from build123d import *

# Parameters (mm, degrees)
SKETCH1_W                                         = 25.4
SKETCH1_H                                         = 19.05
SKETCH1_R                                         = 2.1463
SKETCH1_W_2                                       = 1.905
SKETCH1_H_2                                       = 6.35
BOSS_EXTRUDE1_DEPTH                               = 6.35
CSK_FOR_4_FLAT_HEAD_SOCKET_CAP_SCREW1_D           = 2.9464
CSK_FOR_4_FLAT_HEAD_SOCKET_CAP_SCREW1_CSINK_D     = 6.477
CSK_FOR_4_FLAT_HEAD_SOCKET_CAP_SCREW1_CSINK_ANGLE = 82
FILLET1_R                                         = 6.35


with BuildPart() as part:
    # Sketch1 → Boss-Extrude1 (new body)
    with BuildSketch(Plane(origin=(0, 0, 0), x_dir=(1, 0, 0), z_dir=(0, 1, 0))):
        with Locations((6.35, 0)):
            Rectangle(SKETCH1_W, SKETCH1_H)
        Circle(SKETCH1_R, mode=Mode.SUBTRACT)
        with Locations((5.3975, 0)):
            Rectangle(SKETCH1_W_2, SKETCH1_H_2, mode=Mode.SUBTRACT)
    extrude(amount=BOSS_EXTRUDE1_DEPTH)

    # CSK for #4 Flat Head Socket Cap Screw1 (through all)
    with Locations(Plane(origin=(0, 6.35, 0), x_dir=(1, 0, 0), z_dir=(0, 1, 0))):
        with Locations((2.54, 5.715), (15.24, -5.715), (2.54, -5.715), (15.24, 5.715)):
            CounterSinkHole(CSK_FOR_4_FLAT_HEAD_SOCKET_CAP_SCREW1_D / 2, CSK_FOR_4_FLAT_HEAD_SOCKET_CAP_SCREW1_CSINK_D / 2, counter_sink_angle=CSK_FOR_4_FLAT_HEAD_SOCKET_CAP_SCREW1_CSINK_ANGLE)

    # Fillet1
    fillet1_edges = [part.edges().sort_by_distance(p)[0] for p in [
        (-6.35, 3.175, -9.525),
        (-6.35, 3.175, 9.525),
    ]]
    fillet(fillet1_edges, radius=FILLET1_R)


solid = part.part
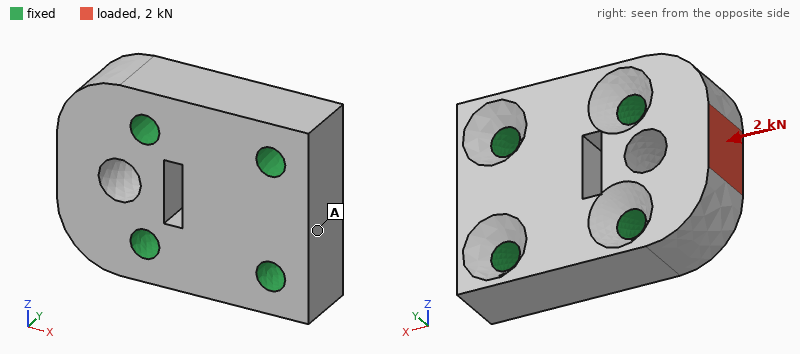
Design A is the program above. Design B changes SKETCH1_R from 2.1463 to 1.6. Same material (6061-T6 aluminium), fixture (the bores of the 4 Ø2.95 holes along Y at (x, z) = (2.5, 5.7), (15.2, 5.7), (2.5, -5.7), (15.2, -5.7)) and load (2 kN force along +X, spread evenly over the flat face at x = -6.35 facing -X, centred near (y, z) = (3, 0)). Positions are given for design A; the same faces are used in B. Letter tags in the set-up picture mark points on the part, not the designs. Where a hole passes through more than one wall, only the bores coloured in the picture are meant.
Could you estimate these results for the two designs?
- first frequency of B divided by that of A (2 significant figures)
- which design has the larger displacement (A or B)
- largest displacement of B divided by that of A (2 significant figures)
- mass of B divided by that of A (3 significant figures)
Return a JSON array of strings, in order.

["1.0", "A", "0.90", "1.02"]
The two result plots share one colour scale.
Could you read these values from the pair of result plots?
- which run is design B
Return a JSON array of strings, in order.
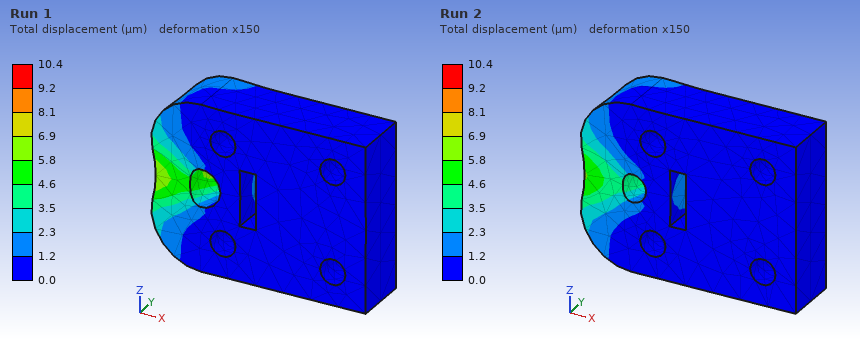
["Run 2"]
